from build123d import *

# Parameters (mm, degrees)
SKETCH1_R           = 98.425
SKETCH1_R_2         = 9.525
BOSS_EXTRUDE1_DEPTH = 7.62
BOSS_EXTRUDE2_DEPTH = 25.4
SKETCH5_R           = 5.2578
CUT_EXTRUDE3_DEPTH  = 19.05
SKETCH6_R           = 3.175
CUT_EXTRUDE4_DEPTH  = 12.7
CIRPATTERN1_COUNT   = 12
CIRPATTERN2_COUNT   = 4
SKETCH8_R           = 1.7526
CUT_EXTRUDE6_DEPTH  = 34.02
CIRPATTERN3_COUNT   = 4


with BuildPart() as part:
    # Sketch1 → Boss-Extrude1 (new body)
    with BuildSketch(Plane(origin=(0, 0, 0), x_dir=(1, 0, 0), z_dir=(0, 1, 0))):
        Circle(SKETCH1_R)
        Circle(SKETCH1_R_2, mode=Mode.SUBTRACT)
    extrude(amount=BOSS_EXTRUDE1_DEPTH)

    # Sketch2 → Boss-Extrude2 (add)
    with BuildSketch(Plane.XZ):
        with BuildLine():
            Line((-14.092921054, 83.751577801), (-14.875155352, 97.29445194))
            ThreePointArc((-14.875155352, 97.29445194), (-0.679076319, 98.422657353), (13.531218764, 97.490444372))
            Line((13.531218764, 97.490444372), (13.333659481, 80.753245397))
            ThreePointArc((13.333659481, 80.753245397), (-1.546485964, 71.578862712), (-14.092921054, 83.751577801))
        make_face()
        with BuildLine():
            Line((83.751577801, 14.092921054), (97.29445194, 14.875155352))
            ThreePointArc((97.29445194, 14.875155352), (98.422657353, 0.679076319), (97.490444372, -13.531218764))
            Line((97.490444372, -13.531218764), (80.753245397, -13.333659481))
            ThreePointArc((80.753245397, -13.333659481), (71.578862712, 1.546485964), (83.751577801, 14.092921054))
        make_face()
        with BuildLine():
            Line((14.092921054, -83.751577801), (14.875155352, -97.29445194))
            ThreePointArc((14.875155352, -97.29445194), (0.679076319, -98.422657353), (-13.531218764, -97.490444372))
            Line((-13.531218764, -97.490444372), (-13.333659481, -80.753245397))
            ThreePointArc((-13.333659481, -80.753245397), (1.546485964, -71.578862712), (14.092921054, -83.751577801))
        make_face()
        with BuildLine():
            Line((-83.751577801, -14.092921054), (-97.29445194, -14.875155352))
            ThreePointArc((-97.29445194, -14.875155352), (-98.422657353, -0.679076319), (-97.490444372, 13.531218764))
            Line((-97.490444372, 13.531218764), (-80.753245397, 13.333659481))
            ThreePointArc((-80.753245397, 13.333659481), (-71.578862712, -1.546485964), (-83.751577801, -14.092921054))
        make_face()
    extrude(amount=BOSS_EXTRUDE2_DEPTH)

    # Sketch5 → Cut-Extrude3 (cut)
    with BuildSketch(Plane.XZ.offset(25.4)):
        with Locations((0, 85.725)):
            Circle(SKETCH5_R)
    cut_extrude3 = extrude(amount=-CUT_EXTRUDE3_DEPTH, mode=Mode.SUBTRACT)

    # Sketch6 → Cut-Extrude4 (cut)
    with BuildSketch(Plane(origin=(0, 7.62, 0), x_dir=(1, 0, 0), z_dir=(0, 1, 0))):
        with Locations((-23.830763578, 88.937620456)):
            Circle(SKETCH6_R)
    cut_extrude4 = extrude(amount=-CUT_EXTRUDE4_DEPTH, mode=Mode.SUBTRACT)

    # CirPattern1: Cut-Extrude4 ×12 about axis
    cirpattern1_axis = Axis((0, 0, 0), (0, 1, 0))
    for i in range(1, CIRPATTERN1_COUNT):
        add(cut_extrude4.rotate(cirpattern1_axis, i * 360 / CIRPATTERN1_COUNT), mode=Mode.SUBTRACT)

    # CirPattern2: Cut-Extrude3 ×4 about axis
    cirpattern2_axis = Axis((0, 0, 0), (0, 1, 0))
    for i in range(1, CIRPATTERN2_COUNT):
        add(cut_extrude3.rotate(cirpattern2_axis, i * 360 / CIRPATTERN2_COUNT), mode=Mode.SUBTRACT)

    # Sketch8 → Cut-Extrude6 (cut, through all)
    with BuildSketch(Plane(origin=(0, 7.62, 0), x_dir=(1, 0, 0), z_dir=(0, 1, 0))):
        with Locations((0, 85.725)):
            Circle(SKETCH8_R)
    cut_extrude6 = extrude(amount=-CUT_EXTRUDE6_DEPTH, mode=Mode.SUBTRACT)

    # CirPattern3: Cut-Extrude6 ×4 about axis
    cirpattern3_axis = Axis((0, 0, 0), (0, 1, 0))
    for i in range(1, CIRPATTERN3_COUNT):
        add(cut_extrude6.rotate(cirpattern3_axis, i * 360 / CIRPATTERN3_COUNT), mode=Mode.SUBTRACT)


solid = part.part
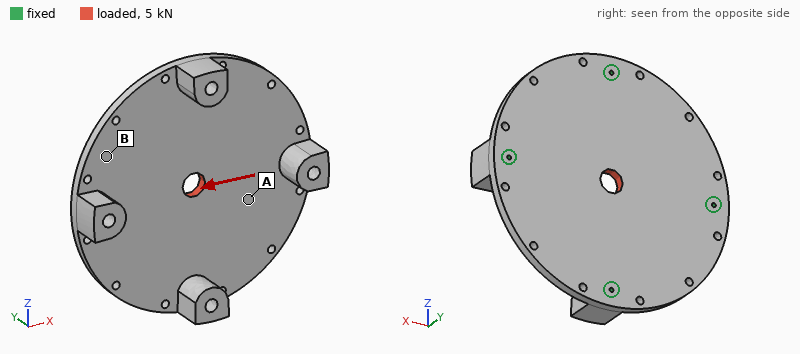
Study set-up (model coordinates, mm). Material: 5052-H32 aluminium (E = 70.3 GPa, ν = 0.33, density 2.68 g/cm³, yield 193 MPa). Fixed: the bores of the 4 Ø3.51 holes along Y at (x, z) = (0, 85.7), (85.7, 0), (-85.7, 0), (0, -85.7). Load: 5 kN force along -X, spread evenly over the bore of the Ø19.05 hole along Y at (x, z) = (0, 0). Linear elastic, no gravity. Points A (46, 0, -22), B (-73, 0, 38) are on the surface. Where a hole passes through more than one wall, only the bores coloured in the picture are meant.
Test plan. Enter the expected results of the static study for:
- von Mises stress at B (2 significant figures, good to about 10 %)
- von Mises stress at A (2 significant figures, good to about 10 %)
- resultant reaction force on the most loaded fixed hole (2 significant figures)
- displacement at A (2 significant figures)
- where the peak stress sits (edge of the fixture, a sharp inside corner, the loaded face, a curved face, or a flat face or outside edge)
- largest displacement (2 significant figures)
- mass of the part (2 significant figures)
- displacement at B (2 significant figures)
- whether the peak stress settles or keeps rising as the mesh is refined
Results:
1.2 MPa
4.1 MPa
1.6 kN
4.0 µm
edge of the fixture
8.1 µm
770 g
3.0 µm
keeps rising
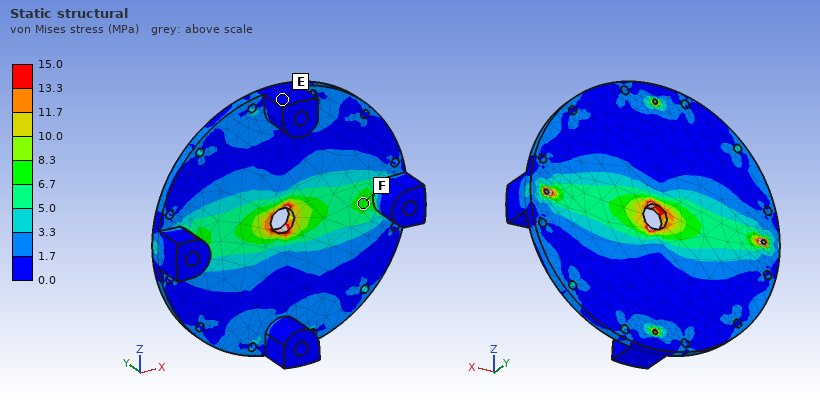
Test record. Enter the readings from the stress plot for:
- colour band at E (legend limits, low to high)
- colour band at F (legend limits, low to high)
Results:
0.0 to 1.7 MPa
6.7 to 8.3 MPa
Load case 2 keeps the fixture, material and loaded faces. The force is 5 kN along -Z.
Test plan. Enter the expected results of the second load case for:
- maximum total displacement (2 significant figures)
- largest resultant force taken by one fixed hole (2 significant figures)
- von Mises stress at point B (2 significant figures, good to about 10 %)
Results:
8.1 µm
1.6 kN
1.8 MPa
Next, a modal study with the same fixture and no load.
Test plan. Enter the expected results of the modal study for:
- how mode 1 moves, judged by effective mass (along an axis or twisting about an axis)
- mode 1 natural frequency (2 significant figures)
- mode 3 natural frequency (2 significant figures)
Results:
along Y
2200 Hz
2700 Hz
